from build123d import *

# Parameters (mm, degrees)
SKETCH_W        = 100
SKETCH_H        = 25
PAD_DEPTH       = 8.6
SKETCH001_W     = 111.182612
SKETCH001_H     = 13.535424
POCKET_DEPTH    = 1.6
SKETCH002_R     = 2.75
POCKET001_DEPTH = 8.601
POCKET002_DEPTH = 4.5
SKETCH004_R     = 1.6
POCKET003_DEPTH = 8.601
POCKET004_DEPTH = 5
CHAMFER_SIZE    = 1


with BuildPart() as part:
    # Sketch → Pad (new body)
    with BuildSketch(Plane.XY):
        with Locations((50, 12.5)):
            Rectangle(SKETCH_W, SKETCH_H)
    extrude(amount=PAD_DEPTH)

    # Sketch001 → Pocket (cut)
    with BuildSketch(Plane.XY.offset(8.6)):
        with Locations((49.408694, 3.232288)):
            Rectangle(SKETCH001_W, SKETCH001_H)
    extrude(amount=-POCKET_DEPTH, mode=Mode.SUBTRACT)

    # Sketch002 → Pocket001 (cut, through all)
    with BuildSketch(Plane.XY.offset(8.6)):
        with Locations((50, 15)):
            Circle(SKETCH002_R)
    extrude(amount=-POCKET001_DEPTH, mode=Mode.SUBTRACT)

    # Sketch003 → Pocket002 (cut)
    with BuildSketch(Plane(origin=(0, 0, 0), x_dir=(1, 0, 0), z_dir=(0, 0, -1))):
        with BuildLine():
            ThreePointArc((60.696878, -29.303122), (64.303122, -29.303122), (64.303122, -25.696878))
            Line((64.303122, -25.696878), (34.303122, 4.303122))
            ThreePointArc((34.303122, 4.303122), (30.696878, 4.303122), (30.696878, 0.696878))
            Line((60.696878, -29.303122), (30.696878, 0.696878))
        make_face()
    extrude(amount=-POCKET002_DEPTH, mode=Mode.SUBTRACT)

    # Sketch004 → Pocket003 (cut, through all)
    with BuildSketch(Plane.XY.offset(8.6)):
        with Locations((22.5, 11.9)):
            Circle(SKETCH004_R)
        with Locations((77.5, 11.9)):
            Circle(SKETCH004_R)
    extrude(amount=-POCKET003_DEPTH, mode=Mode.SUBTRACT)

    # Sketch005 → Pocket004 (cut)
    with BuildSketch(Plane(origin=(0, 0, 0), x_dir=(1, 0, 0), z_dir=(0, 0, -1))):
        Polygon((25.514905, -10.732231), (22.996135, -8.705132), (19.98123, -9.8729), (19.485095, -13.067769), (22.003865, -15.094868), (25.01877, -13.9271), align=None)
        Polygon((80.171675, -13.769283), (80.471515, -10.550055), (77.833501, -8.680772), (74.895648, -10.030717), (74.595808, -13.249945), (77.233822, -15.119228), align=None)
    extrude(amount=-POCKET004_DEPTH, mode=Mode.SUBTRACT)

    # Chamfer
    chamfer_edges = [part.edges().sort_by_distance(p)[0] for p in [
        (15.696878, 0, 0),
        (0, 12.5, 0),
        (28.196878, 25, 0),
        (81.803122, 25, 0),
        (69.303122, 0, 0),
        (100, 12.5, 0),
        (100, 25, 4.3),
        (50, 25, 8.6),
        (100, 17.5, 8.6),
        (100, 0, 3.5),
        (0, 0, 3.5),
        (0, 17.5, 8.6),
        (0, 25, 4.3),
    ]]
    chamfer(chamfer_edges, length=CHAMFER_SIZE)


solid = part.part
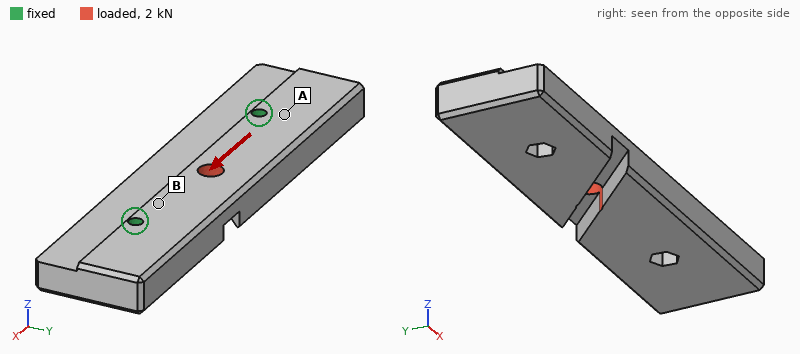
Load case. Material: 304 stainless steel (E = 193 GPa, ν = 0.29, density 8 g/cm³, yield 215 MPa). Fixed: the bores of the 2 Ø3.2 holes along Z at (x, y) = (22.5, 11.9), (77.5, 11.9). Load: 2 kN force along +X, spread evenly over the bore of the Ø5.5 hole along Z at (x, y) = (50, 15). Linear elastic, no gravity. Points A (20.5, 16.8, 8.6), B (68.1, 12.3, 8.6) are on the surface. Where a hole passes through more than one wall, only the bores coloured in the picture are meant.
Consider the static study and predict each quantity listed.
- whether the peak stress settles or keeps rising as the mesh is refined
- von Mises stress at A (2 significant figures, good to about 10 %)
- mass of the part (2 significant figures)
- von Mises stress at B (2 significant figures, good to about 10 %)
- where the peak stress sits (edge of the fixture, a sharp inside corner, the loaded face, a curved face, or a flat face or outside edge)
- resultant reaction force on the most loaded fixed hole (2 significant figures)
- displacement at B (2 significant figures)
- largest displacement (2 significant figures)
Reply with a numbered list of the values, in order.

1. keeps rising
2. 7.2 MPa
3. 150 g
4. 18 MPa
5. edge of the fixture
6. 1.0 kN
7. 0.98 µm
8. 3.1 µm
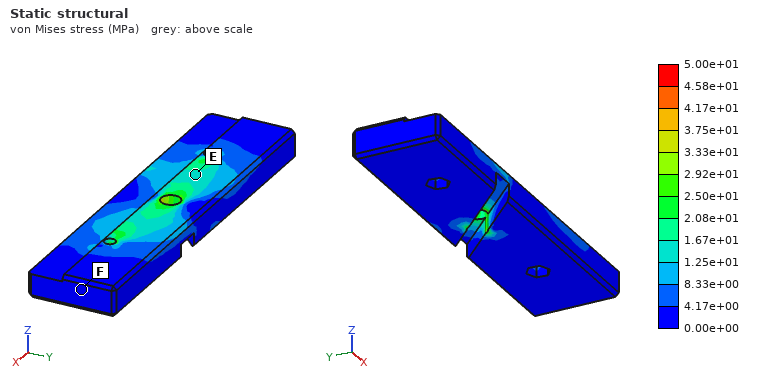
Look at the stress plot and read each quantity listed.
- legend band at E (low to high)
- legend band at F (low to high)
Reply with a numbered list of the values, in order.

1. 1.25e+01 to 1.67e+01 MPa
2. 0.00e+00 to 4.17e+00 MPa
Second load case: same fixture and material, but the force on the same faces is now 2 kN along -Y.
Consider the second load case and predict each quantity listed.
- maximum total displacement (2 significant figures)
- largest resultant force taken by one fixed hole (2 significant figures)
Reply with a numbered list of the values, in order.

1. 10 µm
2. 1.0 kN
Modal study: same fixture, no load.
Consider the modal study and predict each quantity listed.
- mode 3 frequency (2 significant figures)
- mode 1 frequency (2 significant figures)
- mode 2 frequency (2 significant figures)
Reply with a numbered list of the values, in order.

1. 7200 Hz
2. 4600 Hz
3. 5400 Hz
